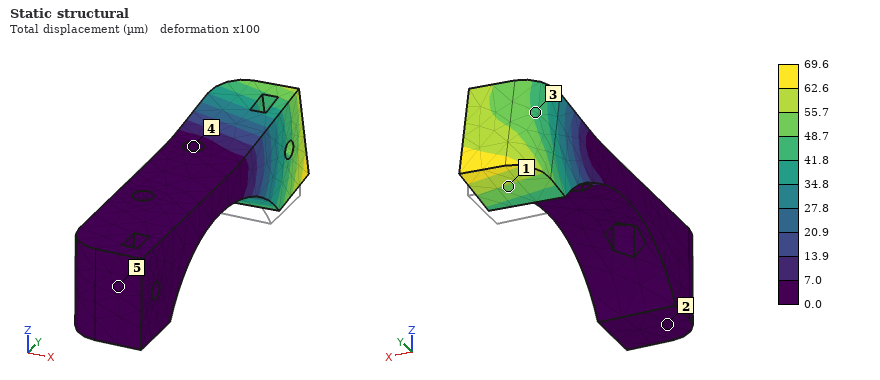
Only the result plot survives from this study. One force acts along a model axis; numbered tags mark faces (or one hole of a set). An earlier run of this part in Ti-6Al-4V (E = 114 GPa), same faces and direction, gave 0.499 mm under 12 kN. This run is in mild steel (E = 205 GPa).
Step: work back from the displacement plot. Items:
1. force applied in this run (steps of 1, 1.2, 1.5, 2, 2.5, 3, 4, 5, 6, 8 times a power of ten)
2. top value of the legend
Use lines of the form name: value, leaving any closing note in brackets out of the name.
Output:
force applied in this run: 3 kN
top value of the legend: 69.6 µm
